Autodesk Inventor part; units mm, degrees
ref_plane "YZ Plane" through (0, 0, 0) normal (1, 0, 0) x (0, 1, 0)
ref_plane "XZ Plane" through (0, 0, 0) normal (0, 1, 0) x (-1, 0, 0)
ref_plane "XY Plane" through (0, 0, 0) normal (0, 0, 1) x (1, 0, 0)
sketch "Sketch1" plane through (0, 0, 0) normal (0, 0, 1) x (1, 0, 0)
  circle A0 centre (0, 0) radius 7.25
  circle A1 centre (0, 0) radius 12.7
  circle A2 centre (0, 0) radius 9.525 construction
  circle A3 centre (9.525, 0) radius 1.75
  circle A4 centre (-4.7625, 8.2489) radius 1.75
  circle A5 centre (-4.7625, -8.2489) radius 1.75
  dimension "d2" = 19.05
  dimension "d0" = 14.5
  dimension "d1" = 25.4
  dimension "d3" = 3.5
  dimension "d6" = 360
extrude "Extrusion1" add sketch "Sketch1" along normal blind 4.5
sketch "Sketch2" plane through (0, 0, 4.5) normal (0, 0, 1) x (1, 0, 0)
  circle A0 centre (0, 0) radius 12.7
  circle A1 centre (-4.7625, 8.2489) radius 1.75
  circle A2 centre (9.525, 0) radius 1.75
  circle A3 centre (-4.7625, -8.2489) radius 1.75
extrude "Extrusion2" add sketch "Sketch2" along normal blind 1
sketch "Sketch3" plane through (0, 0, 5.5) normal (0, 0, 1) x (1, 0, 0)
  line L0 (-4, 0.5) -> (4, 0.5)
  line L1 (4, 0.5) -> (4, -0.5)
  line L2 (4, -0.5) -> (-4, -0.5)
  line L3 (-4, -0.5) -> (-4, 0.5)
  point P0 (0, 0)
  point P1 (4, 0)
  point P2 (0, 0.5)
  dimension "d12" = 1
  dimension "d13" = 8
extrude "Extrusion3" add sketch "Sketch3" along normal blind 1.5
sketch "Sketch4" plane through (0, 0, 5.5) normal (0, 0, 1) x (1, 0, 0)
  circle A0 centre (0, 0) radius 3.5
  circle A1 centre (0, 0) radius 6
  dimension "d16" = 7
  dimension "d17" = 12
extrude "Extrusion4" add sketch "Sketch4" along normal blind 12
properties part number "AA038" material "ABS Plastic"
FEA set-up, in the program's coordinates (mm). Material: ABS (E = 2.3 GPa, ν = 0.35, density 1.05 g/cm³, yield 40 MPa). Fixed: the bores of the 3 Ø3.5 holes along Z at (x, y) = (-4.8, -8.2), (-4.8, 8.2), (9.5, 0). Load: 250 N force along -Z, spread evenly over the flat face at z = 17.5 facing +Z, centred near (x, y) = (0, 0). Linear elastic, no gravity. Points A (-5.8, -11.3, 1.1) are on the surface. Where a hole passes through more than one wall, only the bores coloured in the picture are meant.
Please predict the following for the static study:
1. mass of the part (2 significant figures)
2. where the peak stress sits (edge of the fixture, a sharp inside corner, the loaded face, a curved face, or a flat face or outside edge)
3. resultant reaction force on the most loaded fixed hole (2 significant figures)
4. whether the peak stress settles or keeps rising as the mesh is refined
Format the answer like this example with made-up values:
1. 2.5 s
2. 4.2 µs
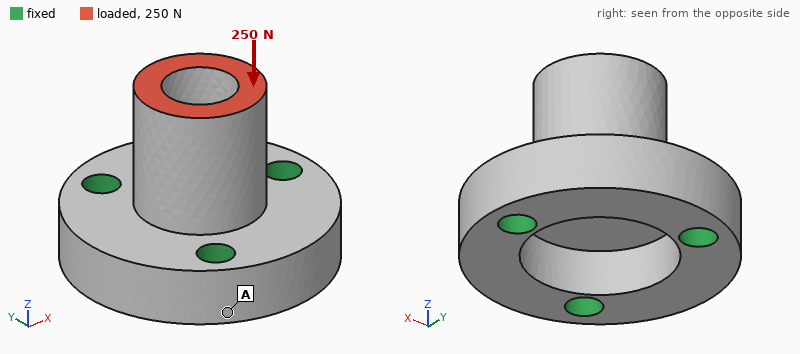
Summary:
1. 2.9 g
2. a sharp inside corner
3. 89 N
4. keeps rising
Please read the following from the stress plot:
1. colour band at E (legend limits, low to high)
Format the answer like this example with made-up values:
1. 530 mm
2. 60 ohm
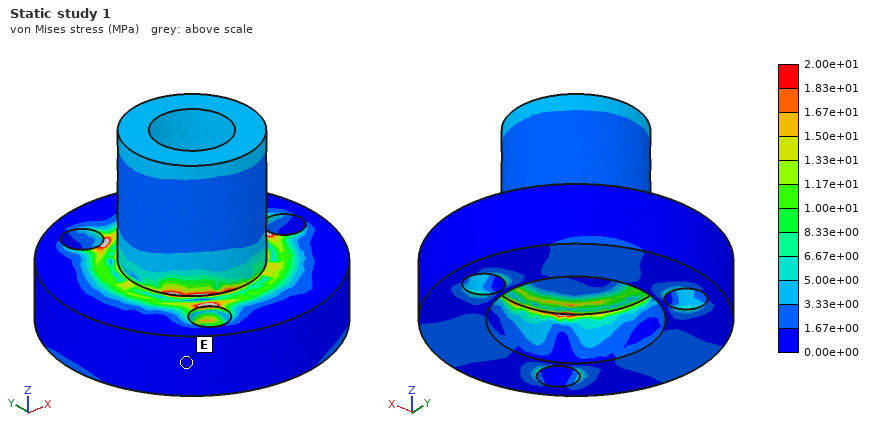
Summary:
1. 0.00e+00 to 1.67e+00 MPa
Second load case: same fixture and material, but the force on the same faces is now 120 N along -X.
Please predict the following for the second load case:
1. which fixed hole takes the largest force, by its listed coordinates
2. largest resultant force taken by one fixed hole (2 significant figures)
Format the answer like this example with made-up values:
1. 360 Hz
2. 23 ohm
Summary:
1. (9.5, 0)
2. 120 N
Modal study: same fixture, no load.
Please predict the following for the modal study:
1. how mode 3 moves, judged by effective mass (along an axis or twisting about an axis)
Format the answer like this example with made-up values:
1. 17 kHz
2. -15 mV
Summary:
1. along Z
